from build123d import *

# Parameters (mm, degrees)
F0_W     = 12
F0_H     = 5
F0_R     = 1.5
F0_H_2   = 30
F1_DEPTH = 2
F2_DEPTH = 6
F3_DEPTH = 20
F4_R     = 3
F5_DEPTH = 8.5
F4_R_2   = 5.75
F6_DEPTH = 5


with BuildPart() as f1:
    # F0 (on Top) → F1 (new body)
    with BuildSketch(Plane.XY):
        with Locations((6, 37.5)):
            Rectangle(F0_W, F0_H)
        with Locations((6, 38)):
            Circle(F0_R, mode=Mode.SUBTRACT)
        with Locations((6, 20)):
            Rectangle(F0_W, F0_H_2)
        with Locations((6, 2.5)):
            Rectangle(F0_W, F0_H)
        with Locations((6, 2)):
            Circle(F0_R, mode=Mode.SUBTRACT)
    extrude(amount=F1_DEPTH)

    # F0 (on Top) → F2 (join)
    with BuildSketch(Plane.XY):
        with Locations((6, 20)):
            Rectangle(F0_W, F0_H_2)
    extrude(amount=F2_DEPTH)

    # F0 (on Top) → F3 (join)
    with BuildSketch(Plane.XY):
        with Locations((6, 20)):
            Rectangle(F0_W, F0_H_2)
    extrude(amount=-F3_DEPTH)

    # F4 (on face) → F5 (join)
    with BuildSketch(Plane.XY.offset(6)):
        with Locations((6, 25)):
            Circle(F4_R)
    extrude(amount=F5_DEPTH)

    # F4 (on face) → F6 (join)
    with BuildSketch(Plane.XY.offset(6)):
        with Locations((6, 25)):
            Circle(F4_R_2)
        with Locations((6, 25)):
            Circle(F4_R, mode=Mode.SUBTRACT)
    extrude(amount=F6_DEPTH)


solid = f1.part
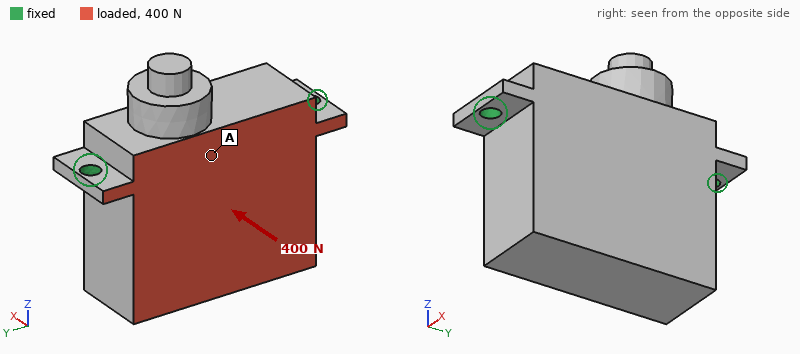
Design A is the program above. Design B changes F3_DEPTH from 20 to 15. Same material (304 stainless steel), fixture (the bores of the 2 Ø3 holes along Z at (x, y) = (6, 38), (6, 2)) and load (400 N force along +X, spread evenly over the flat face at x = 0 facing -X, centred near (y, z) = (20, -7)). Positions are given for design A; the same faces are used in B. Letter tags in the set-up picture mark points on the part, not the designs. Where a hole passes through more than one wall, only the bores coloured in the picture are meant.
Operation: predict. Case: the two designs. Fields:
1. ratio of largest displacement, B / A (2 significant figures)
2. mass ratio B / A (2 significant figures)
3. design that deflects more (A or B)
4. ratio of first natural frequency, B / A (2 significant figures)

0.54
0.82
A
1.4
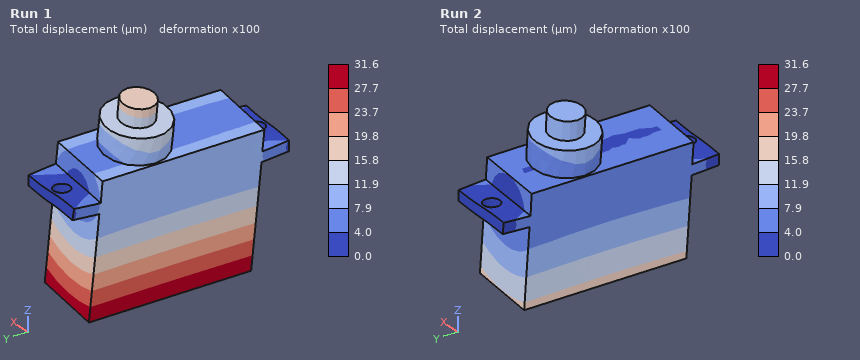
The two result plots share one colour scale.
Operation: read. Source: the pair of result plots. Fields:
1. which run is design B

Run 2
